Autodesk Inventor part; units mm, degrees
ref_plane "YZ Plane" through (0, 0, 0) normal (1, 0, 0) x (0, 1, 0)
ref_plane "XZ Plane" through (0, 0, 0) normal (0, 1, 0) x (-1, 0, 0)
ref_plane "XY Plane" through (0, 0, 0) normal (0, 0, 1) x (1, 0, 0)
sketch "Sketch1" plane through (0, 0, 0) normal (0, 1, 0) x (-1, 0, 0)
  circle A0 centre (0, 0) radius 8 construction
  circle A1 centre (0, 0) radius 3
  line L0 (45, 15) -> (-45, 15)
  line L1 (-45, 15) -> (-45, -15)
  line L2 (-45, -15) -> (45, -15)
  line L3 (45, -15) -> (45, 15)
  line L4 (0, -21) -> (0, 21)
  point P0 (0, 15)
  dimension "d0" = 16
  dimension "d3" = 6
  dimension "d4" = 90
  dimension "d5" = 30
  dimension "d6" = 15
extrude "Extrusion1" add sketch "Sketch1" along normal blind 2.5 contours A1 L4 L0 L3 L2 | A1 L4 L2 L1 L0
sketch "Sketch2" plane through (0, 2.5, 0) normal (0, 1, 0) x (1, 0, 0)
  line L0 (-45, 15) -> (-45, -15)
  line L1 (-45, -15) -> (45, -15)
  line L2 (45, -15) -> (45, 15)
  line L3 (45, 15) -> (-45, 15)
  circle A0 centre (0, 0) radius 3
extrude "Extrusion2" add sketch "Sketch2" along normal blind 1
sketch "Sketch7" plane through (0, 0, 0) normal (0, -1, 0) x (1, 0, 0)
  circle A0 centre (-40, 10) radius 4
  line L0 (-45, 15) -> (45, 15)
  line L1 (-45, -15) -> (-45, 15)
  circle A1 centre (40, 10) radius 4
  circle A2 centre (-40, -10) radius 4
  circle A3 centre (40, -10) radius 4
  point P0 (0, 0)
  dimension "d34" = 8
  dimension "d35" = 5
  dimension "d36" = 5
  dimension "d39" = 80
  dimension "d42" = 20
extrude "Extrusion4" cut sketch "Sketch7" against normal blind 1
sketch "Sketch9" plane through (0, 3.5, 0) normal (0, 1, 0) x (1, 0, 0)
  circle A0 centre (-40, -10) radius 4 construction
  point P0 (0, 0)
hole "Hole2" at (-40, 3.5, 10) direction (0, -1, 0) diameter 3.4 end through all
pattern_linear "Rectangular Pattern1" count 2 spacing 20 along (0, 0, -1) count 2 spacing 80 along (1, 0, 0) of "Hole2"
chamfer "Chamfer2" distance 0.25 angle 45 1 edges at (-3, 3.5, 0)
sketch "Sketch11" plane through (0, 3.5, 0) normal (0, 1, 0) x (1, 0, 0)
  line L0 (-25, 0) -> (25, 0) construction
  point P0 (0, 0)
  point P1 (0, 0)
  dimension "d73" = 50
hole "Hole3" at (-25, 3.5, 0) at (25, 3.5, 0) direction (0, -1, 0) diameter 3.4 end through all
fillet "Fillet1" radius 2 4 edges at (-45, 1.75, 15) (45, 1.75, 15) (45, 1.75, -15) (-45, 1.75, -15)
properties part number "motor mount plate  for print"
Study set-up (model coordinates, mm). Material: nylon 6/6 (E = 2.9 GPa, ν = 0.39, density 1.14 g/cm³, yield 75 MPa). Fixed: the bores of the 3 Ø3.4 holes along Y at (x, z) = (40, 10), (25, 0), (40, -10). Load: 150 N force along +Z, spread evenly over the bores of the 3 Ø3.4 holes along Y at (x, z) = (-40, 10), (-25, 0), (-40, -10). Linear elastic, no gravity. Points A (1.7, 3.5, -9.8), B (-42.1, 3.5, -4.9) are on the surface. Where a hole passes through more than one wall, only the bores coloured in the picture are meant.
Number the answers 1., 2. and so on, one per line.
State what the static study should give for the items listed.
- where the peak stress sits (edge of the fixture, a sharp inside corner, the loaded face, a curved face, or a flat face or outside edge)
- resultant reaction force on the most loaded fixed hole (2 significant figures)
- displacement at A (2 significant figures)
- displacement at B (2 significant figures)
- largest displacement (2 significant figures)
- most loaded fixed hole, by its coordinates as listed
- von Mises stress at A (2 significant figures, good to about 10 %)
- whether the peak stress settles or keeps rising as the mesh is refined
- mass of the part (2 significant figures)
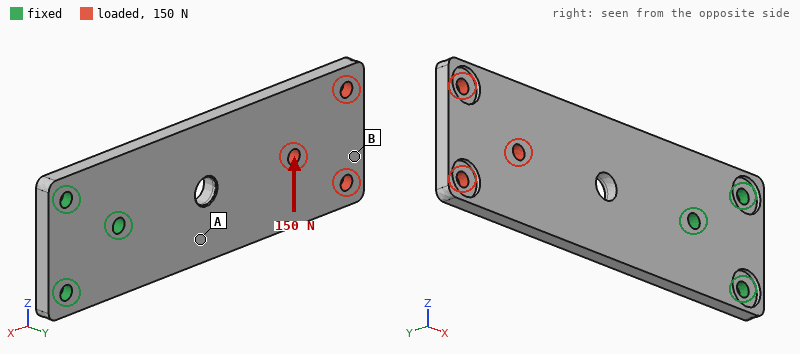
1. edge of the fixture
2. 340 N
3. 0.30 mm
4. 1.0 mm
5. 1.1 mm
6. (25, 0)
7. 7.8 MPa
8. keeps rising
9. 10 g
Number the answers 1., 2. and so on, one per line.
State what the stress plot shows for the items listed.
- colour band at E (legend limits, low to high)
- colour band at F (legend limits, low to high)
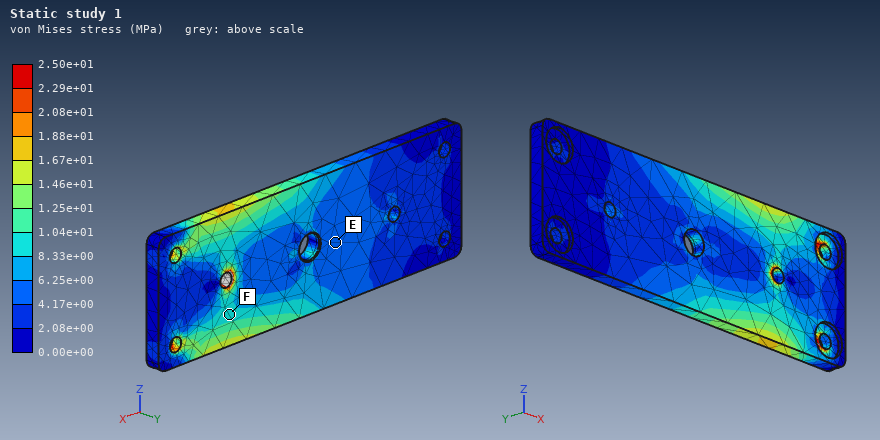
1. 4.17e+00 to 6.25e+00 MPa
2. 8.33e+00 to 1.04e+01 MPa
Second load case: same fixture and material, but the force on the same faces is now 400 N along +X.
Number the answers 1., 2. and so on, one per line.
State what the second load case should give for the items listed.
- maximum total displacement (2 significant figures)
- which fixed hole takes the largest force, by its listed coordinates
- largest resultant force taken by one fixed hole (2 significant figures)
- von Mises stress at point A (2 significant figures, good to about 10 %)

1. 0.98 mm
2. (25, 0)
3. 250 N
4. 6.2 MPa
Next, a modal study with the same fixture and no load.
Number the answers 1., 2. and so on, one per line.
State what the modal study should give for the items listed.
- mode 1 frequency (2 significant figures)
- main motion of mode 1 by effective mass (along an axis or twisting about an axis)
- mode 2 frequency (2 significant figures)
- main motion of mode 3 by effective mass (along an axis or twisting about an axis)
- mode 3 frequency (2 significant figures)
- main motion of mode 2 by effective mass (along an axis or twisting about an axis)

1. 190 Hz
2. along Y
3. 770 Hz
4. along Z
5. 1100 Hz
6. twisting about X
